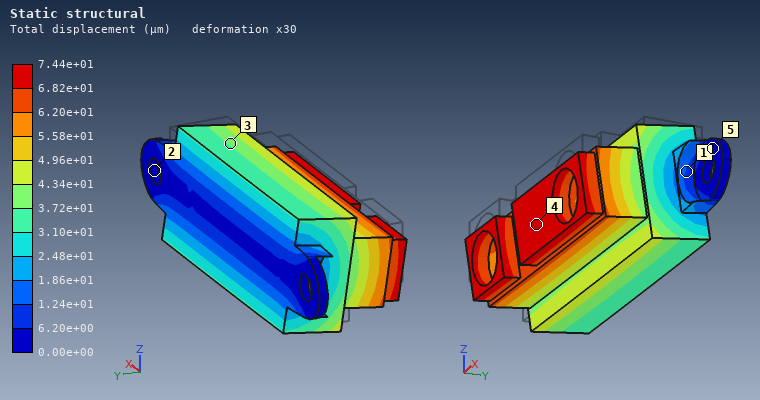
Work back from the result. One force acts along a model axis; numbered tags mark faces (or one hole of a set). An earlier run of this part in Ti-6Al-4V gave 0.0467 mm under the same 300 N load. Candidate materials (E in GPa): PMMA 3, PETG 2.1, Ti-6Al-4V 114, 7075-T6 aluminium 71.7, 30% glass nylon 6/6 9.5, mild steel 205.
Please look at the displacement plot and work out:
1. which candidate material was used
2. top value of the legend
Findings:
7075-T6 aluminium
7.44e+01 µm
